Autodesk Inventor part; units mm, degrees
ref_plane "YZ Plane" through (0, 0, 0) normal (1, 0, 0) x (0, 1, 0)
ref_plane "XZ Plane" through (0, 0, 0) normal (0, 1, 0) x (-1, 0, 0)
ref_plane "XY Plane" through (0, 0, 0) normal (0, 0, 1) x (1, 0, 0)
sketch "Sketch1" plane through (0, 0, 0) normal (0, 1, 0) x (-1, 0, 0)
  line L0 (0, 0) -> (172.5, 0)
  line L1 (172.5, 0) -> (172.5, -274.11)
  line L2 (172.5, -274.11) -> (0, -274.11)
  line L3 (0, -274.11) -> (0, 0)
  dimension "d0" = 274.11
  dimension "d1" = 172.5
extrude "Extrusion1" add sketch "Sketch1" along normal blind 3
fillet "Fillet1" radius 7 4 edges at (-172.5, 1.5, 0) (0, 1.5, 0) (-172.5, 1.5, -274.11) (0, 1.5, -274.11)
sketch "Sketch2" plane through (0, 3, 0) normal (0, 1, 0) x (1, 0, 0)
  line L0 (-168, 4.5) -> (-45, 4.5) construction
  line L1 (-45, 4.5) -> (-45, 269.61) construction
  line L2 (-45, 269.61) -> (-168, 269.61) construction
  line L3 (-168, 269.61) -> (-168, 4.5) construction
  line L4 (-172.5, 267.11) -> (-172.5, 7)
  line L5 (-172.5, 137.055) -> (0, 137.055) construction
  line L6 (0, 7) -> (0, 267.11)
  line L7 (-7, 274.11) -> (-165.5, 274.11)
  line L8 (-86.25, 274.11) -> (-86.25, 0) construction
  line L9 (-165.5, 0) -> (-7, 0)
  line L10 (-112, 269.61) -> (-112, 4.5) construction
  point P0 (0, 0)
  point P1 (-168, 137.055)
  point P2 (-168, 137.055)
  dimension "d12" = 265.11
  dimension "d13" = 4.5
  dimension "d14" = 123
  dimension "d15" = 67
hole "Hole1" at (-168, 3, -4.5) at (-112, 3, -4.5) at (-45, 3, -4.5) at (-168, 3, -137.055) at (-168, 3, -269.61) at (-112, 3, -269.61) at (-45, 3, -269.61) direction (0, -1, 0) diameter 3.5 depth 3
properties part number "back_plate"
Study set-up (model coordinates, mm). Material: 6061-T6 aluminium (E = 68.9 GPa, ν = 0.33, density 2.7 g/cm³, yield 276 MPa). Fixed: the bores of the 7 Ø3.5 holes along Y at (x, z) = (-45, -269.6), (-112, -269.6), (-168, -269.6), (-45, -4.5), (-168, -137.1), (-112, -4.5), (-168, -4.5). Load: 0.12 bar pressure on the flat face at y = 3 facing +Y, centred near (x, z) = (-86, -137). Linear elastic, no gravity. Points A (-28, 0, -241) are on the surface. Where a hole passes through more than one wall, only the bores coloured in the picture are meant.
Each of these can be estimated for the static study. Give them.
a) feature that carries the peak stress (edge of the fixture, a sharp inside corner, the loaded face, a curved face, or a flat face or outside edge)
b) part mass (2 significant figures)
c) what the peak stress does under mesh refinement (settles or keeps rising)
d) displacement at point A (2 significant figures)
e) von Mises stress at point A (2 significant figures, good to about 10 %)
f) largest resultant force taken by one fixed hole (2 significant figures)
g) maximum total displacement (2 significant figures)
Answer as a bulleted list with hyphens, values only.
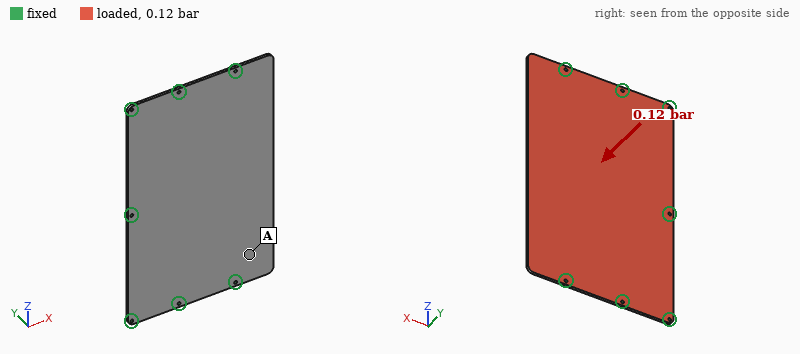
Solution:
- edge of the fixture
- 380 g
- keeps rising
- 0.31 mm
- 11 MPa
- 150 N
- 1.4 mm
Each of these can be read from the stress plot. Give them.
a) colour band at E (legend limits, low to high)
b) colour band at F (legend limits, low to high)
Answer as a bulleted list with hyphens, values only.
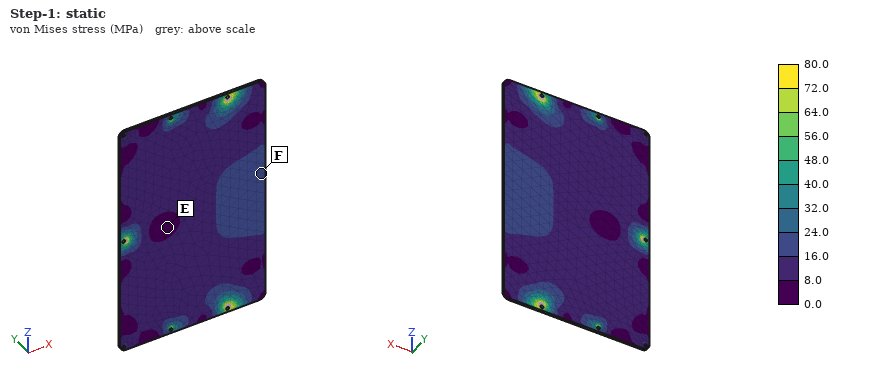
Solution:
- 0.0 to 8.0 MPa
- 16.0 to 24.0 MPa
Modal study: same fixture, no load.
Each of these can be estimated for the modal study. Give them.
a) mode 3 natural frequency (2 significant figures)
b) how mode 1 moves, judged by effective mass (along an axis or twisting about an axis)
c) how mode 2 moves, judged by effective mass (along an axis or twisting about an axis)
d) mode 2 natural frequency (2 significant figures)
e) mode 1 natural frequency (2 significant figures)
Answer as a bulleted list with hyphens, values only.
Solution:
- 570 Hz
- along Y
- twisting about X
- 540 Hz
- 220 Hz
